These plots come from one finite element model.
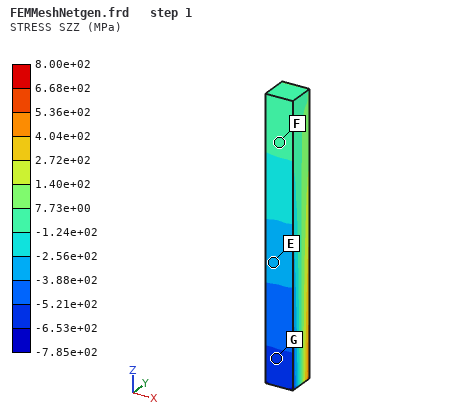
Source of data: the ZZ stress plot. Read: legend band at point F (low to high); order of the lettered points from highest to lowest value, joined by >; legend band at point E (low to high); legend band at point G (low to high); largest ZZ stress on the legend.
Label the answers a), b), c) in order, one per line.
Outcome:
a) -1.24e+02 to 7.73e+00 MPa
b) F > E > G
c) -3.88e+02 to -2.56e+02 MPa
d) -6.53e+02 to -5.21e+02 MPa
e) 8.00e+02 MPa
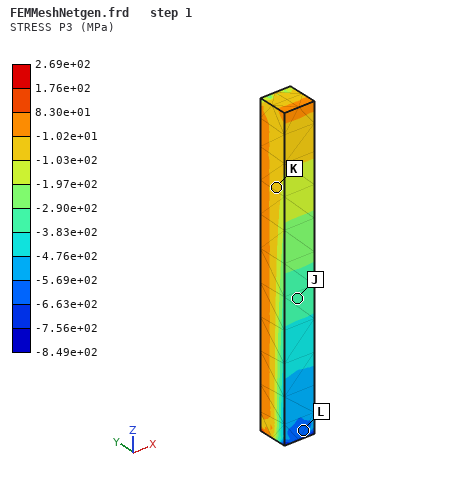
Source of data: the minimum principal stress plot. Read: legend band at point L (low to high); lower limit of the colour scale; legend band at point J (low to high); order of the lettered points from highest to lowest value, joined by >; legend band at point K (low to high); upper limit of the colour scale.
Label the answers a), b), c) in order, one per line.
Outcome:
a) -6.63e+02 to -5.69e+02 MPa
b) -8.49e+02 MPa
c) -3.83e+02 to -2.90e+02 MPa
d) K > J > L
e) -1.03e+02 to -1.02e+01 MPa
f) 2.69e+02 MPa
